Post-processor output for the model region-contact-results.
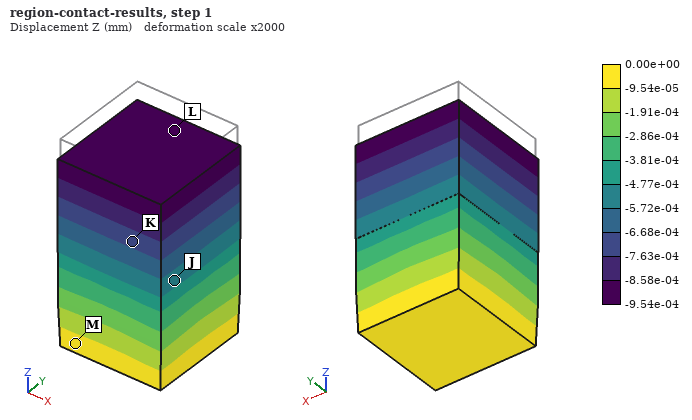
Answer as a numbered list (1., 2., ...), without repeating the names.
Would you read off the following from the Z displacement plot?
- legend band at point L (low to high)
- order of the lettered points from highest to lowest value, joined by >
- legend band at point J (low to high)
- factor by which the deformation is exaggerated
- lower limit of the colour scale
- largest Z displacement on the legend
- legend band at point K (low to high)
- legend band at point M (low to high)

1. -9.54e-04 to -8.58e-04 mm
2. M > J > K > L
3. -5.72e-04 to -4.77e-04 mm
4. 2000
5. -9.54e-04 mm
6. 0.00e+00 mm
7. -7.63e-04 to -6.68e-04 mm
8. -9.54e-05 to 0.00e+00 mm
